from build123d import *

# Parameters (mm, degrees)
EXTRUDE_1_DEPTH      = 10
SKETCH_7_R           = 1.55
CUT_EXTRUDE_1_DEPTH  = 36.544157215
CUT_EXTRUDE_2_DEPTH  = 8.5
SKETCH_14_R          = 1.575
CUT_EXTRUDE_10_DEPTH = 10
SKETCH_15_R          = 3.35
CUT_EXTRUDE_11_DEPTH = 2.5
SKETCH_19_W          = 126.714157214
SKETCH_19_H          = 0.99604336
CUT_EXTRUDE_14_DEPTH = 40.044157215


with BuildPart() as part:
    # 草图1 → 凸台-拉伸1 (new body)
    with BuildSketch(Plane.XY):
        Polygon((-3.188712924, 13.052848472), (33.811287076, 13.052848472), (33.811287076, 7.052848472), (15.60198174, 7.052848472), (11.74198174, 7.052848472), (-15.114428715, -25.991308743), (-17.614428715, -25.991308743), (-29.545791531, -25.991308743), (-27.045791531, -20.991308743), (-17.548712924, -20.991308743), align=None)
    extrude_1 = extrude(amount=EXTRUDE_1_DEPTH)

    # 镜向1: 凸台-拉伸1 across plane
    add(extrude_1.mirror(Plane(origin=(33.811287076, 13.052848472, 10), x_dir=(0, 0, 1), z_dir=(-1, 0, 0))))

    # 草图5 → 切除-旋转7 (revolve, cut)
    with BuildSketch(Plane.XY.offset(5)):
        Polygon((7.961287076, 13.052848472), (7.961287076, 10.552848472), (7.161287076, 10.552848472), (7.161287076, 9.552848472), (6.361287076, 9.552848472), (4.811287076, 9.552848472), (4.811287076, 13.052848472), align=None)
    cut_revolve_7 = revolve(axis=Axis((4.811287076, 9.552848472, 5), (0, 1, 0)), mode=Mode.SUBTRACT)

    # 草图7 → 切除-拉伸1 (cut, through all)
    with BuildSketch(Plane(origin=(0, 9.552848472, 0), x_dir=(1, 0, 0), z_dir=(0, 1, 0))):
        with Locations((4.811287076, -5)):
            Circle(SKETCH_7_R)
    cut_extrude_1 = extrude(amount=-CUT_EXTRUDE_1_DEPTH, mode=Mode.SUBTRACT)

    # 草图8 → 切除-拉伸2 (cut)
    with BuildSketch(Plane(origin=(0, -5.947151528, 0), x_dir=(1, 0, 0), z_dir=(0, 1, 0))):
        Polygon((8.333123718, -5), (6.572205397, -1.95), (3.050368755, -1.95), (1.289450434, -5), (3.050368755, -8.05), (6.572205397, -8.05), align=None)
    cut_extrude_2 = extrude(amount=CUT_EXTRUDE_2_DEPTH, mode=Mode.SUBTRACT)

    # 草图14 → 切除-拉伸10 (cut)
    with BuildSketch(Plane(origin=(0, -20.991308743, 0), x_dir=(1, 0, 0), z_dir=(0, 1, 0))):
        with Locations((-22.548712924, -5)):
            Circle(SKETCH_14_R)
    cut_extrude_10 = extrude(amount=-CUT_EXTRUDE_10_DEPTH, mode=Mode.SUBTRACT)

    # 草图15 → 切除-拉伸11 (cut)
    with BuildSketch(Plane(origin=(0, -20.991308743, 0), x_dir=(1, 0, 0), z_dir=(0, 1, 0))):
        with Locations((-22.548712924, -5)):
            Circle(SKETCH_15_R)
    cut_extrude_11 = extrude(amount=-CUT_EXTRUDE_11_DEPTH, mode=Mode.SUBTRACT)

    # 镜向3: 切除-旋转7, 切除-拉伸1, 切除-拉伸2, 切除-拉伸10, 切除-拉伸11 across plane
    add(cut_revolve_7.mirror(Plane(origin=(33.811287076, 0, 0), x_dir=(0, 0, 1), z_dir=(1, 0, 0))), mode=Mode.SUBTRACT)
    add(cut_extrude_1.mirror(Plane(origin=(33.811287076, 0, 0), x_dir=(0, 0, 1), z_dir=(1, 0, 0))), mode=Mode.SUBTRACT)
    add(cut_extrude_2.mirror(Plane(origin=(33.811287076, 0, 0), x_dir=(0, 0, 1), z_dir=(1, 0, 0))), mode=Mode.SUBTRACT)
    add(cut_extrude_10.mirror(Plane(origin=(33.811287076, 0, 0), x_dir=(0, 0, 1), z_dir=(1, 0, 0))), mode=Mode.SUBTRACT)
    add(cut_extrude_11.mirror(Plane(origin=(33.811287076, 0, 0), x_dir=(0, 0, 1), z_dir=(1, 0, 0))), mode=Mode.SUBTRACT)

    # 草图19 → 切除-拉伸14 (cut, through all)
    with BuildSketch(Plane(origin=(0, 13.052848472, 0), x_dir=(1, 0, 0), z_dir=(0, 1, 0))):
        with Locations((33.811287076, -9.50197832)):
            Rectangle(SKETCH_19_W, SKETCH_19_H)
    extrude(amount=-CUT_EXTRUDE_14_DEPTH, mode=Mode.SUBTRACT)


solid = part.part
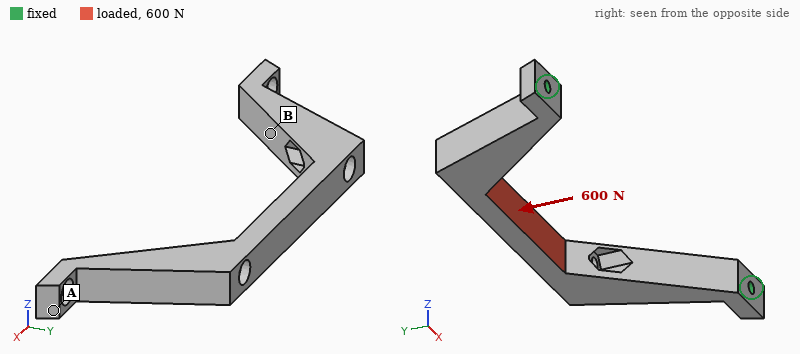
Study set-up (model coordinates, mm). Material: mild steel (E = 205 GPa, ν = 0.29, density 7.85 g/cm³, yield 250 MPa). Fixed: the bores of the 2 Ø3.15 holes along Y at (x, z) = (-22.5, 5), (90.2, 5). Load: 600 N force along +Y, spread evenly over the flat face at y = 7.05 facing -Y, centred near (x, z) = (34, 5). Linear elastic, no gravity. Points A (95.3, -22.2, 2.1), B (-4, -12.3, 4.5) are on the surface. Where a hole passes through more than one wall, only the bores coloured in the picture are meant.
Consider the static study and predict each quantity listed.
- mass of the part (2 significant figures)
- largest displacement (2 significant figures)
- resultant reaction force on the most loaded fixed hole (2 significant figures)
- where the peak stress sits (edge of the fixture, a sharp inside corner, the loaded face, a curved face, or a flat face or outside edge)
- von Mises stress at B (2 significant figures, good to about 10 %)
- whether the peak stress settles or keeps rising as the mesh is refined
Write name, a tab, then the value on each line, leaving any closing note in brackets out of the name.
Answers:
mass of the part	85 g
largest displacement	16 µm
resultant reaction force on the most loaded fixed hole	440 N
where the peak stress sits	edge of the fixture
von Mises stress at B	13 MPa
whether the peak stress settles or keeps rising as the mesh is refined	keeps rising
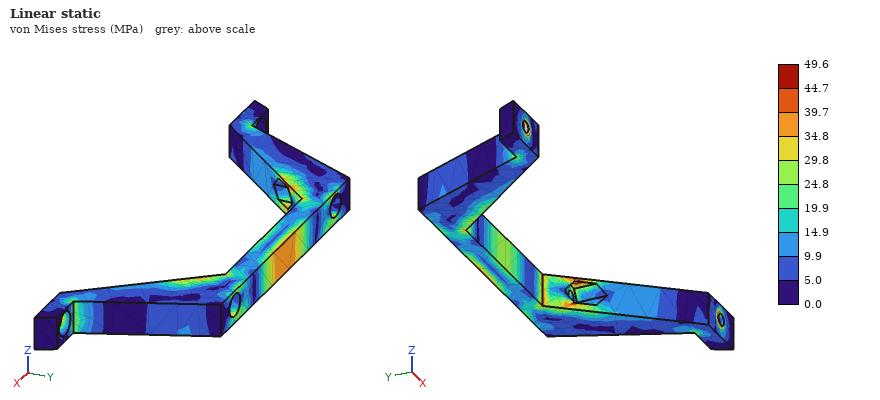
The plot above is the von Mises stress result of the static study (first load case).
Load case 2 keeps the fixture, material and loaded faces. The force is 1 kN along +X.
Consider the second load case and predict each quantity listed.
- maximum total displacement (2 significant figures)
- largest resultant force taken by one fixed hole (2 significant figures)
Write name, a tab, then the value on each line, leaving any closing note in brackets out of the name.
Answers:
maximum total displacement	63 µm
largest resultant force taken by one fixed hole	560 N
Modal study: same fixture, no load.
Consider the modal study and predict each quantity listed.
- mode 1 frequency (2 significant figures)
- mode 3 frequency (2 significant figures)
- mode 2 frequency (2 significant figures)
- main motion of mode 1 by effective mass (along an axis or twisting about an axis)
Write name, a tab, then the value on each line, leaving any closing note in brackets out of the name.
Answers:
mode 1 frequency	1100 Hz
mode 3 frequency	2800 Hz
mode 2 frequency	2700 Hz
main motion of mode 1 by effective mass	along Z
